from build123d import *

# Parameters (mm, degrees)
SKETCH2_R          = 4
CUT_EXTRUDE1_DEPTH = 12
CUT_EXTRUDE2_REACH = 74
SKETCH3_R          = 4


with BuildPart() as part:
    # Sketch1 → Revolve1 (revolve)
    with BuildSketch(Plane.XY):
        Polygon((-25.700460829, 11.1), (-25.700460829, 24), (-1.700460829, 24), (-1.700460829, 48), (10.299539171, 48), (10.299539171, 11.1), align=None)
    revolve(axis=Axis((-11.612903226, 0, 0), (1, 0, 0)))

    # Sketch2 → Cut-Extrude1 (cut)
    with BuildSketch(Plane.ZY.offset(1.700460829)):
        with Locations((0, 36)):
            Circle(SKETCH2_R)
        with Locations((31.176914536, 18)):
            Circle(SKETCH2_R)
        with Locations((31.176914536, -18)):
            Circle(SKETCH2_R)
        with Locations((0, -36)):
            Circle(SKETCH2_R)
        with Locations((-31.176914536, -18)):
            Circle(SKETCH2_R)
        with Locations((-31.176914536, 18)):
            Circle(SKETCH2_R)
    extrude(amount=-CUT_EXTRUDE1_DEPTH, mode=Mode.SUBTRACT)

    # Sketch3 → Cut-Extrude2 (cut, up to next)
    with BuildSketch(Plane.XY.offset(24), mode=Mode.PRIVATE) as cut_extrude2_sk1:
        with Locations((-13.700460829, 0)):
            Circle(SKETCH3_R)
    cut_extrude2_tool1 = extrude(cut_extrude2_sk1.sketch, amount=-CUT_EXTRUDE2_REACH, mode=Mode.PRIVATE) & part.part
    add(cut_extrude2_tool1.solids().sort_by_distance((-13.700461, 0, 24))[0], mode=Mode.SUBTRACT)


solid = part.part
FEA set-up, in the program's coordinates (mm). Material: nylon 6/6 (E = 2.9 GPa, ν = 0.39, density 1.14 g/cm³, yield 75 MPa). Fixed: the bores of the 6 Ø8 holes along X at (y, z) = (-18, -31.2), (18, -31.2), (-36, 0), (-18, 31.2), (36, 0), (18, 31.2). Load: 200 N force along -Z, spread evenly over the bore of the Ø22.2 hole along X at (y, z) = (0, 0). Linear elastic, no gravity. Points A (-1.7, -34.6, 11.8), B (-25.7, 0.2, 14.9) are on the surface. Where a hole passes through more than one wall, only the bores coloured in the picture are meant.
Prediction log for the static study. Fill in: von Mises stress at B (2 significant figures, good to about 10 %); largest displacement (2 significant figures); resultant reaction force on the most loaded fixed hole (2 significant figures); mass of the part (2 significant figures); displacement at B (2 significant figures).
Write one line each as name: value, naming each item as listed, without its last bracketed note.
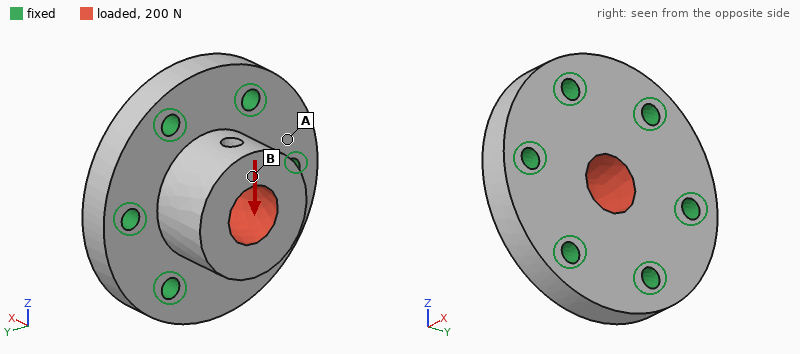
von Mises stress at B: 0.13 MPa
largest displacement: 5.1 µm
resultant reaction force on the most loaded fixed hole: 50 N
mass of the part: 130 g
displacement at B: 5.0 µm
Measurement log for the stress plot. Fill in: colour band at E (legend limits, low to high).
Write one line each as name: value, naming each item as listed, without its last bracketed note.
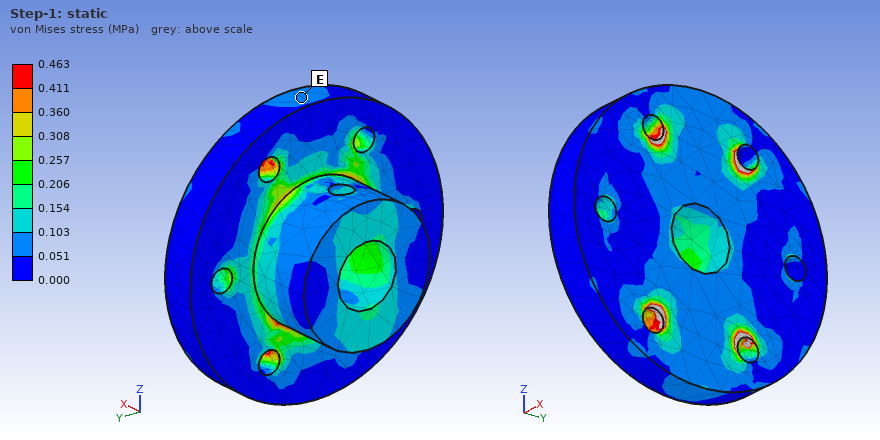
colour band at E: 0.051 to 0.103 MPa
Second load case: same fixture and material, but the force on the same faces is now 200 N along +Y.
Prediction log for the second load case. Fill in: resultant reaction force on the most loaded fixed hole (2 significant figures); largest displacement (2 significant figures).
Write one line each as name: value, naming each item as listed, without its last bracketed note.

resultant reaction force on the most loaded fixed hole: 57 N
largest displacement: 5.2 µm
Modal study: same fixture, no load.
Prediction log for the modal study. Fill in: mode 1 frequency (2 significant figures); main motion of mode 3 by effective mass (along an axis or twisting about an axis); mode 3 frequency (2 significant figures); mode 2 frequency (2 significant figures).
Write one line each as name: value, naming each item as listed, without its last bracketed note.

mode 1 frequency: 4800 Hz
main motion of mode 3 by effective mass: along X
mode 3 frequency: 5000 Hz
mode 2 frequency: 4800 Hz
